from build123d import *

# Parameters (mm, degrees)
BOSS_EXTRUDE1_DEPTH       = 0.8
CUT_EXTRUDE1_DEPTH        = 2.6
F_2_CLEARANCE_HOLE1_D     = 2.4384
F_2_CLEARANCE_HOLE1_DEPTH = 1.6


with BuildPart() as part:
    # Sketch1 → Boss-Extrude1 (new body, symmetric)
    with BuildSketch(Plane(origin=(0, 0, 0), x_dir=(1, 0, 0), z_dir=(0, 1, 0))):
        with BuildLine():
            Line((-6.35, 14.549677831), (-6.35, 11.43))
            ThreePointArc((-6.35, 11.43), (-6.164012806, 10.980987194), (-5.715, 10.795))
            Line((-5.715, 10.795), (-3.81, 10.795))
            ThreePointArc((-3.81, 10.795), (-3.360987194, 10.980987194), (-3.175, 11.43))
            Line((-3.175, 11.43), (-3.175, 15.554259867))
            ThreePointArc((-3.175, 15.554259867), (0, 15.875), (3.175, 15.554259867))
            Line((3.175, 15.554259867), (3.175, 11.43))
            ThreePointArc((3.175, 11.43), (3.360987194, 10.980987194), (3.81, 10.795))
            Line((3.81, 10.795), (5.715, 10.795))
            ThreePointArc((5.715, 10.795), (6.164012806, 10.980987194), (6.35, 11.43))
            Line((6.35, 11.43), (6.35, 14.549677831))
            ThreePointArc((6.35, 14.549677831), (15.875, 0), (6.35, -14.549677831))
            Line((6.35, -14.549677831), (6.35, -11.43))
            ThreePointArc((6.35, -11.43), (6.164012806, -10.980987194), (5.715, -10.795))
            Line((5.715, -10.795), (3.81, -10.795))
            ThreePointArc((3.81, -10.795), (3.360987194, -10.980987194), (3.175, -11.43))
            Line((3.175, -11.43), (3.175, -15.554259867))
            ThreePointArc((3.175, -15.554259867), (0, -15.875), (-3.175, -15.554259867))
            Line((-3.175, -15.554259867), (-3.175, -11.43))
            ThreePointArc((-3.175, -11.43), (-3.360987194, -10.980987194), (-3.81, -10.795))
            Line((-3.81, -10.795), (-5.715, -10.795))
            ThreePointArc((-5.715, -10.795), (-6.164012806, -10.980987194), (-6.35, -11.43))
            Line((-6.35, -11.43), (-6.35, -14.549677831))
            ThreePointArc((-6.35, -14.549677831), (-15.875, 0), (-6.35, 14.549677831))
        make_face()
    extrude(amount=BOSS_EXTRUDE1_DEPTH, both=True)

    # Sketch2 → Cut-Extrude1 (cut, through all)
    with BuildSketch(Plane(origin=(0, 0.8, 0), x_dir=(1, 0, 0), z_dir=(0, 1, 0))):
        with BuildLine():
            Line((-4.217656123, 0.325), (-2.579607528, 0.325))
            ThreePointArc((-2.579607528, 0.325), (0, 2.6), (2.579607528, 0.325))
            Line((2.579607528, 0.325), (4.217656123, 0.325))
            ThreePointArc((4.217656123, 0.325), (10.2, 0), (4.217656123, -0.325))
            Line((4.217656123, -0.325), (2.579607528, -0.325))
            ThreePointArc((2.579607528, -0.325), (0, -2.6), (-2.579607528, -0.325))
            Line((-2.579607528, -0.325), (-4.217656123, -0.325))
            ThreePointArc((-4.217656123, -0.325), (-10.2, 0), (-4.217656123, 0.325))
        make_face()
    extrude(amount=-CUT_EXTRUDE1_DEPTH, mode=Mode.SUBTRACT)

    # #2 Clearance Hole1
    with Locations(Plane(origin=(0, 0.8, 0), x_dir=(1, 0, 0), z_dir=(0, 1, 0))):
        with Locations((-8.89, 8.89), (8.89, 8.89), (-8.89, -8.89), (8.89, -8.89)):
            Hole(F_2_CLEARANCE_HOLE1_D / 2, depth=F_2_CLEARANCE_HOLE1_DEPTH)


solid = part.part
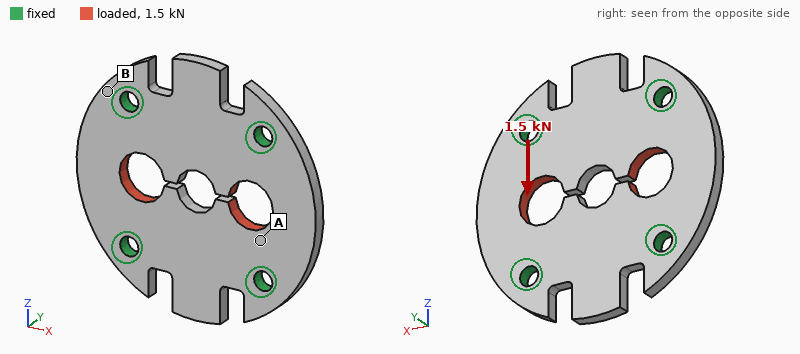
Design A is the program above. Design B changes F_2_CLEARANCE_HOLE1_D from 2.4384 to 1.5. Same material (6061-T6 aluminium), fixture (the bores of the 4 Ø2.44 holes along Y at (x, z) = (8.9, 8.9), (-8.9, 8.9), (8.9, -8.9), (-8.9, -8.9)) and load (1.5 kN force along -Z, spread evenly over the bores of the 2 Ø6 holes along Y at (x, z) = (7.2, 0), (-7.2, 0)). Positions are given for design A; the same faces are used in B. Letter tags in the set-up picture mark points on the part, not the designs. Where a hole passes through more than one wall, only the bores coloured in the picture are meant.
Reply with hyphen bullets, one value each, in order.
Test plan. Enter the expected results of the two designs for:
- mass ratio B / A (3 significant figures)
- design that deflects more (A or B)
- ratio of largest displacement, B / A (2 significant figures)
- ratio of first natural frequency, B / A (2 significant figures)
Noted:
- 1.02
- B
- 1.1
- 0.93
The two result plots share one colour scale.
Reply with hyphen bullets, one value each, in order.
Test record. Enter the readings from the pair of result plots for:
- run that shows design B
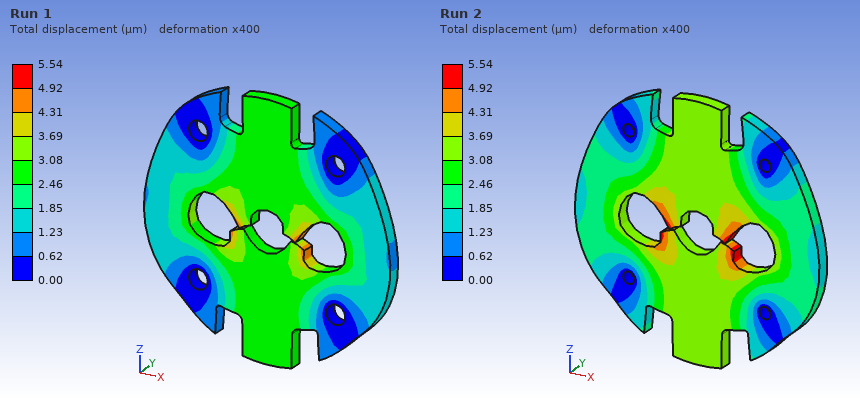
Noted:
- Run 2
